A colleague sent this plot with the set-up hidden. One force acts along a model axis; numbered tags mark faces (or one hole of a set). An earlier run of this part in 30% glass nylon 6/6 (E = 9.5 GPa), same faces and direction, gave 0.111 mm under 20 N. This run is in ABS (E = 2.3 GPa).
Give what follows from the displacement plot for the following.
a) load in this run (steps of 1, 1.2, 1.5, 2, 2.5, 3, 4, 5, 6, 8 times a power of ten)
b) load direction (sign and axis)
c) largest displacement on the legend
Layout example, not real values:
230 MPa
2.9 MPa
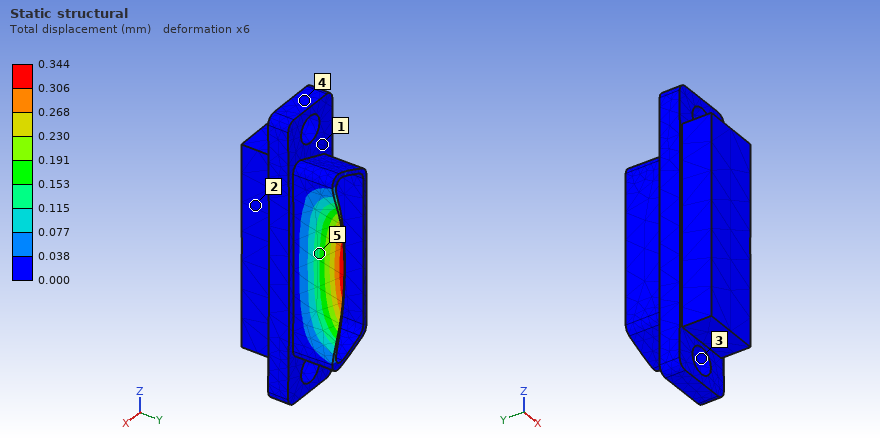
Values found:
15 N
-X
0.344 mm
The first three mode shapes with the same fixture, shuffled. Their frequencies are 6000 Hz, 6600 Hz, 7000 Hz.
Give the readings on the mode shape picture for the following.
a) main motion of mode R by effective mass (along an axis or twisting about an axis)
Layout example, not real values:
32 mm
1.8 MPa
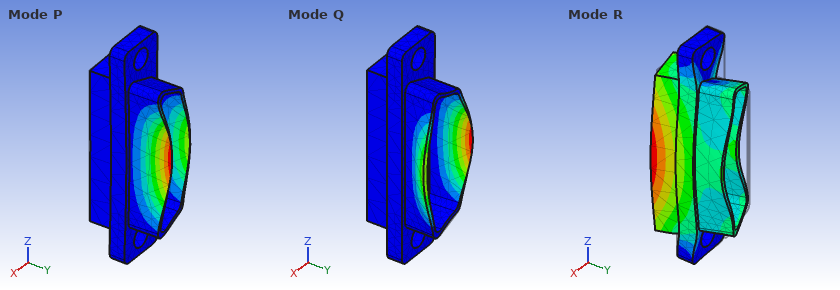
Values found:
along X
